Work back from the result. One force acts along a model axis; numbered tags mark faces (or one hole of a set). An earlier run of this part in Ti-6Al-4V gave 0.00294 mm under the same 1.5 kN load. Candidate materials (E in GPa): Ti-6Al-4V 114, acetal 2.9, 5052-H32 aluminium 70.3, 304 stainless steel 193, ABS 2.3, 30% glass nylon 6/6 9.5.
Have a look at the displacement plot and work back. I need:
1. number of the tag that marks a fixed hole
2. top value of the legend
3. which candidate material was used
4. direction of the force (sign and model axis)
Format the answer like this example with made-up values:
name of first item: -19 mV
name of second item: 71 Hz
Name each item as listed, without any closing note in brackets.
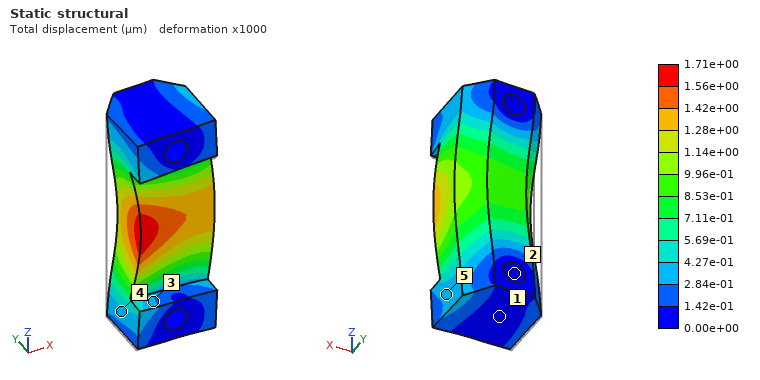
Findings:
number of the tag that marks a fixed hole: 2
top value of the legend: 1.71e+00 µm
which candidate material was used: 304 stainless steel
direction of the force: +X
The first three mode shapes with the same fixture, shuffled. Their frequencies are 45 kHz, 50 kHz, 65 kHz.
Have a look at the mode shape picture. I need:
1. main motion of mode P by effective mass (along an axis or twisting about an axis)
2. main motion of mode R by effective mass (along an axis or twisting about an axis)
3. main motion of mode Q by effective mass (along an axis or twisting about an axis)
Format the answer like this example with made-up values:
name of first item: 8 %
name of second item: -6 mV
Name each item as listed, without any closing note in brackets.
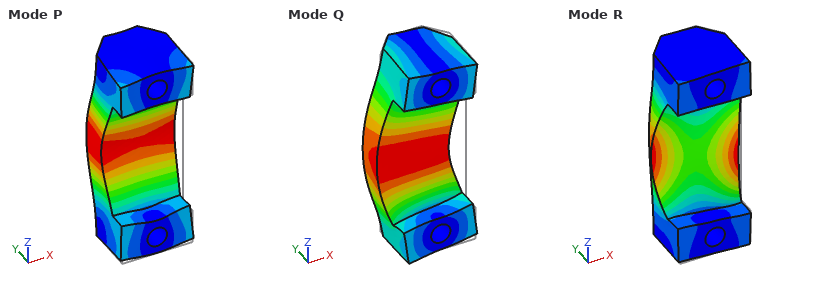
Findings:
main motion of mode P by effective mass: along Y
main motion of mode R by effective mass: twisting about Z
main motion of mode Q by effective mass: along X
